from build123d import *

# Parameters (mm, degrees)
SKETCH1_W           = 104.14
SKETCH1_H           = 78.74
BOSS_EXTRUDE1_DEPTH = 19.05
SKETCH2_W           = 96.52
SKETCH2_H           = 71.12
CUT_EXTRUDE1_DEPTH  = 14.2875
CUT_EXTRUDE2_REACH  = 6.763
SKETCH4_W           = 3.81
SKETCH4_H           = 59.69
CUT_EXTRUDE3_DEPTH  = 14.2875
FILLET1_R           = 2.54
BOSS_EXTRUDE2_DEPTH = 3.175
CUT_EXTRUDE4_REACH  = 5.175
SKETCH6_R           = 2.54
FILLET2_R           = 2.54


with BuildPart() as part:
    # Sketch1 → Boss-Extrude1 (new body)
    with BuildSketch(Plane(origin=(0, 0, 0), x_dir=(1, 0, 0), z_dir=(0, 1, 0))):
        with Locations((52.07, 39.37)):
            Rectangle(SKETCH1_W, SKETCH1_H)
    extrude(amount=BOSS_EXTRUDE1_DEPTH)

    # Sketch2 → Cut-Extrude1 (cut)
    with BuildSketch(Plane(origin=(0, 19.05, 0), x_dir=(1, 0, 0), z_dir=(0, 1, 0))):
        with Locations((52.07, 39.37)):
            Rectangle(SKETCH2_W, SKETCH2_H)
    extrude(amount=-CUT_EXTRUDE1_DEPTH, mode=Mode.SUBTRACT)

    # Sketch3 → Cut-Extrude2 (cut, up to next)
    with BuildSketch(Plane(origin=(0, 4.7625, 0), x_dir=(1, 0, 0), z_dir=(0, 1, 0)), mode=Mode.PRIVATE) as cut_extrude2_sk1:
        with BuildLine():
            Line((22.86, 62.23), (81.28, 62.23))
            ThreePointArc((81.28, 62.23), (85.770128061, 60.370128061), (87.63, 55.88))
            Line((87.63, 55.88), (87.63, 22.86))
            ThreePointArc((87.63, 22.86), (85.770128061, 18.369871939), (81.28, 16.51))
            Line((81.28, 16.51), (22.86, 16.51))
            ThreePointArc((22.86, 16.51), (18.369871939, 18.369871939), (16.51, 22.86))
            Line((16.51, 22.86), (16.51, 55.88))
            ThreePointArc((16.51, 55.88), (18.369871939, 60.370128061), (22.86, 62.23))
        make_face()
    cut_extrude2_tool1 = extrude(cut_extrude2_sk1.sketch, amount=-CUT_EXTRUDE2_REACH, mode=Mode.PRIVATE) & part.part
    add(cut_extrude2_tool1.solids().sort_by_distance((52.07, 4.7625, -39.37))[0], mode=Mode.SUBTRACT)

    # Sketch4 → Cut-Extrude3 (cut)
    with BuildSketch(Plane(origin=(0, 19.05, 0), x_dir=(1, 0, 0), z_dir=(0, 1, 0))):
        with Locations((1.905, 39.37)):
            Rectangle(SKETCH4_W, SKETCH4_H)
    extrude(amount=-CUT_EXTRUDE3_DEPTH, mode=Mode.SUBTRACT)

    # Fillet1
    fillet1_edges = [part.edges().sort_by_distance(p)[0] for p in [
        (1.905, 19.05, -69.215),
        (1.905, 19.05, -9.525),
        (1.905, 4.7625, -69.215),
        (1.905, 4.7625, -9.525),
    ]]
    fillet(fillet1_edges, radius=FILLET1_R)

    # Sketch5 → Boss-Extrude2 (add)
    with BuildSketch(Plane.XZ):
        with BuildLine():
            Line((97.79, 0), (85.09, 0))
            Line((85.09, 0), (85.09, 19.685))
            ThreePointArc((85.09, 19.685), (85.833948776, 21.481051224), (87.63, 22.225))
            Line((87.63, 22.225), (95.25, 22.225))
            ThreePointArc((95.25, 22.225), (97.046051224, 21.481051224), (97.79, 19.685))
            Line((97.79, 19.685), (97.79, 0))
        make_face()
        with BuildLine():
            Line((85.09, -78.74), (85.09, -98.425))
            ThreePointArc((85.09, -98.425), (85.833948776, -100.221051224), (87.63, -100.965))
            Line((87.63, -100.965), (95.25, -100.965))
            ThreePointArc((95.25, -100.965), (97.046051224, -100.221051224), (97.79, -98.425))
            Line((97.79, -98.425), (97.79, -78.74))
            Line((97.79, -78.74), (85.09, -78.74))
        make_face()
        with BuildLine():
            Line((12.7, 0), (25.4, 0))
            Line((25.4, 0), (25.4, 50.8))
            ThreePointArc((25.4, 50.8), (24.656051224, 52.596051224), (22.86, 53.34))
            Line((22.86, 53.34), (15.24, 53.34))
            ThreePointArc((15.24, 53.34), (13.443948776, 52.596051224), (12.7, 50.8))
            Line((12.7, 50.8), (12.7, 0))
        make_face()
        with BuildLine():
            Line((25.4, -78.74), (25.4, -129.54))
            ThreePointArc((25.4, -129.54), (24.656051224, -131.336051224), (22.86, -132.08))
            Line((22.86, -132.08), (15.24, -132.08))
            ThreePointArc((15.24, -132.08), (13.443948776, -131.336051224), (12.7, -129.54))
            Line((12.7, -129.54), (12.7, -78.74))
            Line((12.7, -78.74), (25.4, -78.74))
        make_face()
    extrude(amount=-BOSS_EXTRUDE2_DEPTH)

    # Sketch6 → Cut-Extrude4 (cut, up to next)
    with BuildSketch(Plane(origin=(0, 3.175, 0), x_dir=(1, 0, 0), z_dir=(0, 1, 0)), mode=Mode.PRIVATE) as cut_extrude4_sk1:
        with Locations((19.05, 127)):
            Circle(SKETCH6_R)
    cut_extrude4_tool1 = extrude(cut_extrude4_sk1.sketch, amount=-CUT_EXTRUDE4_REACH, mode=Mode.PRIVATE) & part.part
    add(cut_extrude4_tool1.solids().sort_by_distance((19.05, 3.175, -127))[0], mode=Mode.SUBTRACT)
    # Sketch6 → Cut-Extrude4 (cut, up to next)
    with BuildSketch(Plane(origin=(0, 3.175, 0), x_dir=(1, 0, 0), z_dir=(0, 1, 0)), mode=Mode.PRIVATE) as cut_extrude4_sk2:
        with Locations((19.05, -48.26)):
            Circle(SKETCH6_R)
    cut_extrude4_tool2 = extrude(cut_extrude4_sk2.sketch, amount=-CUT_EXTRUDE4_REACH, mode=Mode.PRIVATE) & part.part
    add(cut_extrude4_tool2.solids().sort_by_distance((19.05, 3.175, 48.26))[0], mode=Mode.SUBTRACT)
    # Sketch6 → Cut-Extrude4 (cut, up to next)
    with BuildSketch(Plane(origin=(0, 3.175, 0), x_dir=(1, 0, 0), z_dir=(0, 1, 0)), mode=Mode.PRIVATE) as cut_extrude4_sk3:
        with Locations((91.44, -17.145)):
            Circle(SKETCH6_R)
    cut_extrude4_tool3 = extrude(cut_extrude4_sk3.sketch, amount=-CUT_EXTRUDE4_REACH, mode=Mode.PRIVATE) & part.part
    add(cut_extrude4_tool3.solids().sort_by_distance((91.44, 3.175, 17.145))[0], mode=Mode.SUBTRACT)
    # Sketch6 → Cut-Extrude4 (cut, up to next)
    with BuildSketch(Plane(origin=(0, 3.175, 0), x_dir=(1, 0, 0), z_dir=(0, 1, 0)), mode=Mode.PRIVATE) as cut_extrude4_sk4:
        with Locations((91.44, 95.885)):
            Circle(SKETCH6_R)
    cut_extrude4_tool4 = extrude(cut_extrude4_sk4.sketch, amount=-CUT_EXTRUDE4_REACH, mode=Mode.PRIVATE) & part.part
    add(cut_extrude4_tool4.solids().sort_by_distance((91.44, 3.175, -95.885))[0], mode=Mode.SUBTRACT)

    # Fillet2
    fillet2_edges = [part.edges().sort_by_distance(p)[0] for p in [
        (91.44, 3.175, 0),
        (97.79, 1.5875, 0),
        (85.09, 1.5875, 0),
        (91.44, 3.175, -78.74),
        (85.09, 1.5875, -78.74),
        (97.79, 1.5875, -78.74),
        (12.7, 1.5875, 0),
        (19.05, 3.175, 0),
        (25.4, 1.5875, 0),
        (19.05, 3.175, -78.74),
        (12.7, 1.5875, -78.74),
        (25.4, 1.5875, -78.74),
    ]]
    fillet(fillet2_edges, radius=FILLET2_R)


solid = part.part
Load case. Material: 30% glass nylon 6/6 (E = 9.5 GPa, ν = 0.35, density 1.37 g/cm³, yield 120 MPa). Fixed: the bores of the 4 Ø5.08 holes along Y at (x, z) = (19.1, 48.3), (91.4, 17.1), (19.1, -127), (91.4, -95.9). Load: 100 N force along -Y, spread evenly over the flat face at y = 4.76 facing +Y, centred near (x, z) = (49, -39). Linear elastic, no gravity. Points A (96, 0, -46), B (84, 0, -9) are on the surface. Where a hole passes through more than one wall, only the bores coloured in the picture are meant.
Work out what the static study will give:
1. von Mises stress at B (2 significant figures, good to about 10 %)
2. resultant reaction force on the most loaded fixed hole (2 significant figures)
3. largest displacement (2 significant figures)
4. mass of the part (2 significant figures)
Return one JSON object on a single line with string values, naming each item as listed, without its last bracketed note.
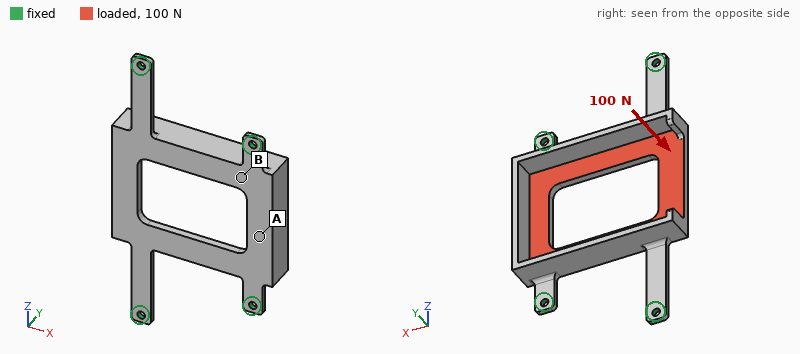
{"von Mises stress at B": "4.1 MPa", "resultant reaction force on the most loaded fixed hole": "46 N", "largest displacement": "1.3 mm", "mass of the part": "62 g"}
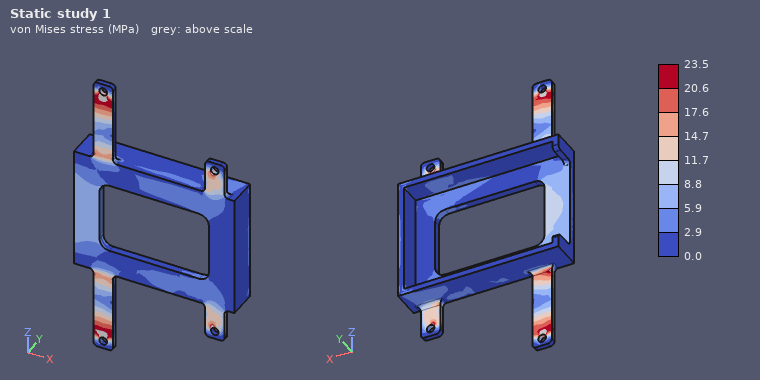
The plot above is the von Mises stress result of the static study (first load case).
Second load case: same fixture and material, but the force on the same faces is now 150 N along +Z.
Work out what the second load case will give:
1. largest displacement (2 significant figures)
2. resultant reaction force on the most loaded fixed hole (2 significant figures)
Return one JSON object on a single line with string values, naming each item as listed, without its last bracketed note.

{"largest displacement": "28 µm", "resultant reaction force on the most loaded fixed hole": "40 N"}
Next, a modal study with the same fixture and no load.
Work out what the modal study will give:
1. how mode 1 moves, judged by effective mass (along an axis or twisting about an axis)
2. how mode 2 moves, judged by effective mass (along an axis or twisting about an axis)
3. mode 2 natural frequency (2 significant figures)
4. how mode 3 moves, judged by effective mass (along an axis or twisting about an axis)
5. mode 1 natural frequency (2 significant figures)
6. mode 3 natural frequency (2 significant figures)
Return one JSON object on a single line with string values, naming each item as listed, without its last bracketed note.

{"how mode 1 moves, judged by effective mass": "along Y", "how mode 2 moves, judged by effective mass": "twisting about X", "mode 2 natural frequency": "590 Hz", "how mode 3 moves, judged by effective mass": "along Y", "mode 1 natural frequency": "250 Hz", "mode 3 natural frequency": "1000 Hz"}
